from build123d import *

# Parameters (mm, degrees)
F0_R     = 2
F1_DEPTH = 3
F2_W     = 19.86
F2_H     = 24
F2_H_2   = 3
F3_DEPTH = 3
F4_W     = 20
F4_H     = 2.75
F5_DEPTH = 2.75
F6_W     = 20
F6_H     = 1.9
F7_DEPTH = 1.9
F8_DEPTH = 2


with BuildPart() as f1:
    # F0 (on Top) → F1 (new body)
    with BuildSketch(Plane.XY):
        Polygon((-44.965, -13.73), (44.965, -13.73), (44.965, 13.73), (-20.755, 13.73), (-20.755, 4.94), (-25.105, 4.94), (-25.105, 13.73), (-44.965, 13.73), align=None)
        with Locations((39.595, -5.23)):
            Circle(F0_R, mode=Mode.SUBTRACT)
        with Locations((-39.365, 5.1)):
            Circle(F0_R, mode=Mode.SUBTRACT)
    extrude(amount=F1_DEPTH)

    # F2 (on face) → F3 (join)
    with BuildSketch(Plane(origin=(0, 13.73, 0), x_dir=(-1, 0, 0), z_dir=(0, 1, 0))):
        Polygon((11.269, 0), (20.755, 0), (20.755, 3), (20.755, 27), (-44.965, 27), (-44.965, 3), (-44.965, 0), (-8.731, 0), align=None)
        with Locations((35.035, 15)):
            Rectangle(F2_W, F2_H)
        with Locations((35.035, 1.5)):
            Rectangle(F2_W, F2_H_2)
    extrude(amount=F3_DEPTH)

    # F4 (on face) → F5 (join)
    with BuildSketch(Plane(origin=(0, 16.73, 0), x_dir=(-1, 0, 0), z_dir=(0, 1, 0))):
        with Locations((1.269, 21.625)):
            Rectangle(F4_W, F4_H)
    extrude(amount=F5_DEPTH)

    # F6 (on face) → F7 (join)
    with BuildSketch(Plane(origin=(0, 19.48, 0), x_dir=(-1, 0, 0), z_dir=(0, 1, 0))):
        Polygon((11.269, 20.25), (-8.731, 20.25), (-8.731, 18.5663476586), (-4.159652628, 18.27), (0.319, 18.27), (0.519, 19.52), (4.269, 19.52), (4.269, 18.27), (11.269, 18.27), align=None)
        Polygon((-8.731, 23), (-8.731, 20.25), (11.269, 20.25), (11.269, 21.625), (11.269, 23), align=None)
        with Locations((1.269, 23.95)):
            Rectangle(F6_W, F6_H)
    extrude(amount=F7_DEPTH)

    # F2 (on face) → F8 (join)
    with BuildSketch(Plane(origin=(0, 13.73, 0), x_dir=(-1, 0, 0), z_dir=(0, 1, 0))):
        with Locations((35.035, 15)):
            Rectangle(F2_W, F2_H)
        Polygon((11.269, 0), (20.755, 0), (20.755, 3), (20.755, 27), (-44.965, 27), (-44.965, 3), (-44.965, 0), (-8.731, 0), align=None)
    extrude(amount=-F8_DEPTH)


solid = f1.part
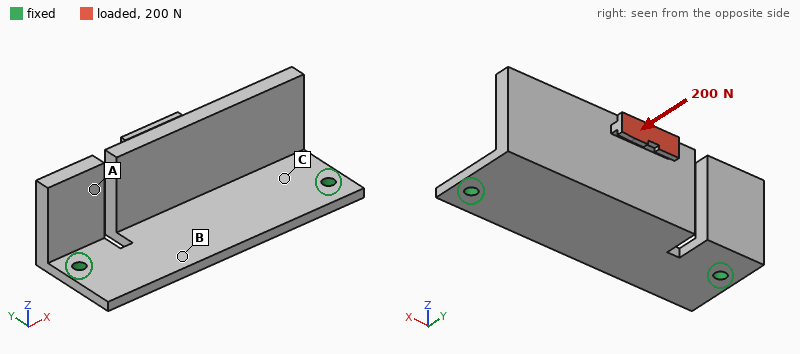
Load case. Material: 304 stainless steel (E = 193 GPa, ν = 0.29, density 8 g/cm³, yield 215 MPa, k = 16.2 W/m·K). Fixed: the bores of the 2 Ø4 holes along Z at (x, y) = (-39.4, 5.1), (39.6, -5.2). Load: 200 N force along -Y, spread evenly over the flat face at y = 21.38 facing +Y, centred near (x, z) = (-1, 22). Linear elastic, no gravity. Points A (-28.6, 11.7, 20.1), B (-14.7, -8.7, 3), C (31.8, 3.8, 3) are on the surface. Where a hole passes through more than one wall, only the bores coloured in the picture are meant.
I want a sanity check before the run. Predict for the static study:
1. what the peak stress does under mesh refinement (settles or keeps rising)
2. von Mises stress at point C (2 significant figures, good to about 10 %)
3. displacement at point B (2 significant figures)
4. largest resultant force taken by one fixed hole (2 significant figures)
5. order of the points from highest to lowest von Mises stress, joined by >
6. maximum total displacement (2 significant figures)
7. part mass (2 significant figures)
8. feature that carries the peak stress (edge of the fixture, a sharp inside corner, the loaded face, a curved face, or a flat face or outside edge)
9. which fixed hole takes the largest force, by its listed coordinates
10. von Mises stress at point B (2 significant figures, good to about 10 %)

keeps rising
49 MPa
0.025 mm
110 N
C > B > A
0.13 mm
150 g
edge of the fixture
(-39.4, 5.1)
19 MPa
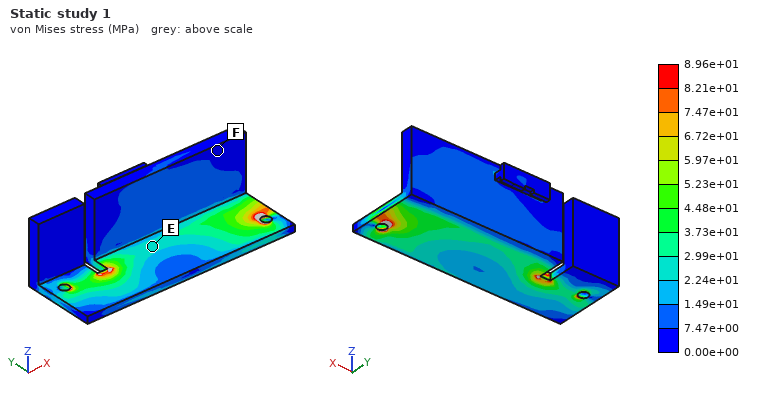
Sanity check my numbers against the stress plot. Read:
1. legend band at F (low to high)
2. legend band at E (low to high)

0.00e+00 to 7.47e+00 MPa
2.24e+01 to 2.99e+01 MPa
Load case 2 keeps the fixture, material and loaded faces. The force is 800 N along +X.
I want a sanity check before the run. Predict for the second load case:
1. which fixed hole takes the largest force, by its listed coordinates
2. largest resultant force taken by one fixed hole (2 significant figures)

(39.6, -5.2)
740 N
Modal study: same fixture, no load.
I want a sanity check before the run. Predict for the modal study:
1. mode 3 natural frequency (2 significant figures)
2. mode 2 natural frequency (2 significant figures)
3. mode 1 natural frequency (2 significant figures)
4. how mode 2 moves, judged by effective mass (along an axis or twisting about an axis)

2200 Hz
1900 Hz
930 Hz
along Z
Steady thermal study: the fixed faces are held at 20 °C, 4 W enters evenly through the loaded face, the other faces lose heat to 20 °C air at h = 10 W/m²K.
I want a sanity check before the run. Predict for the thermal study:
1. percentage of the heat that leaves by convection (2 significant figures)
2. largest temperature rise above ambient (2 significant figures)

55 %
71 K
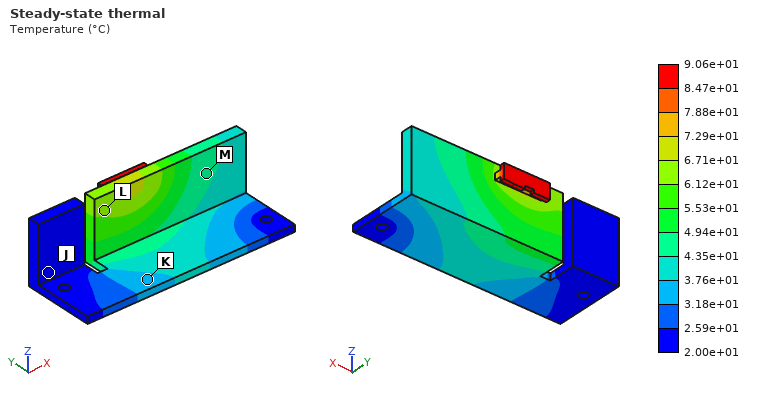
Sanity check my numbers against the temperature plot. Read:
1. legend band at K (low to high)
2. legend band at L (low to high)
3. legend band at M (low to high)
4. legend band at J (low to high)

3.18e+01 to 3.76e+01 °C
6.12e+01 to 6.71e+01 °C
4.35e+01 to 4.94e+01 °C
2.00e+01 to 2.59e+01 °C
